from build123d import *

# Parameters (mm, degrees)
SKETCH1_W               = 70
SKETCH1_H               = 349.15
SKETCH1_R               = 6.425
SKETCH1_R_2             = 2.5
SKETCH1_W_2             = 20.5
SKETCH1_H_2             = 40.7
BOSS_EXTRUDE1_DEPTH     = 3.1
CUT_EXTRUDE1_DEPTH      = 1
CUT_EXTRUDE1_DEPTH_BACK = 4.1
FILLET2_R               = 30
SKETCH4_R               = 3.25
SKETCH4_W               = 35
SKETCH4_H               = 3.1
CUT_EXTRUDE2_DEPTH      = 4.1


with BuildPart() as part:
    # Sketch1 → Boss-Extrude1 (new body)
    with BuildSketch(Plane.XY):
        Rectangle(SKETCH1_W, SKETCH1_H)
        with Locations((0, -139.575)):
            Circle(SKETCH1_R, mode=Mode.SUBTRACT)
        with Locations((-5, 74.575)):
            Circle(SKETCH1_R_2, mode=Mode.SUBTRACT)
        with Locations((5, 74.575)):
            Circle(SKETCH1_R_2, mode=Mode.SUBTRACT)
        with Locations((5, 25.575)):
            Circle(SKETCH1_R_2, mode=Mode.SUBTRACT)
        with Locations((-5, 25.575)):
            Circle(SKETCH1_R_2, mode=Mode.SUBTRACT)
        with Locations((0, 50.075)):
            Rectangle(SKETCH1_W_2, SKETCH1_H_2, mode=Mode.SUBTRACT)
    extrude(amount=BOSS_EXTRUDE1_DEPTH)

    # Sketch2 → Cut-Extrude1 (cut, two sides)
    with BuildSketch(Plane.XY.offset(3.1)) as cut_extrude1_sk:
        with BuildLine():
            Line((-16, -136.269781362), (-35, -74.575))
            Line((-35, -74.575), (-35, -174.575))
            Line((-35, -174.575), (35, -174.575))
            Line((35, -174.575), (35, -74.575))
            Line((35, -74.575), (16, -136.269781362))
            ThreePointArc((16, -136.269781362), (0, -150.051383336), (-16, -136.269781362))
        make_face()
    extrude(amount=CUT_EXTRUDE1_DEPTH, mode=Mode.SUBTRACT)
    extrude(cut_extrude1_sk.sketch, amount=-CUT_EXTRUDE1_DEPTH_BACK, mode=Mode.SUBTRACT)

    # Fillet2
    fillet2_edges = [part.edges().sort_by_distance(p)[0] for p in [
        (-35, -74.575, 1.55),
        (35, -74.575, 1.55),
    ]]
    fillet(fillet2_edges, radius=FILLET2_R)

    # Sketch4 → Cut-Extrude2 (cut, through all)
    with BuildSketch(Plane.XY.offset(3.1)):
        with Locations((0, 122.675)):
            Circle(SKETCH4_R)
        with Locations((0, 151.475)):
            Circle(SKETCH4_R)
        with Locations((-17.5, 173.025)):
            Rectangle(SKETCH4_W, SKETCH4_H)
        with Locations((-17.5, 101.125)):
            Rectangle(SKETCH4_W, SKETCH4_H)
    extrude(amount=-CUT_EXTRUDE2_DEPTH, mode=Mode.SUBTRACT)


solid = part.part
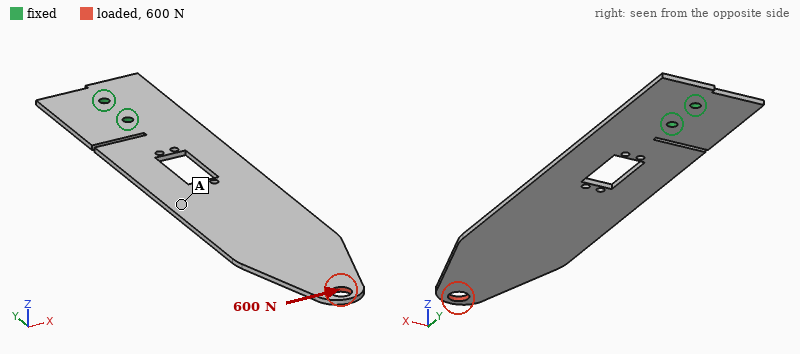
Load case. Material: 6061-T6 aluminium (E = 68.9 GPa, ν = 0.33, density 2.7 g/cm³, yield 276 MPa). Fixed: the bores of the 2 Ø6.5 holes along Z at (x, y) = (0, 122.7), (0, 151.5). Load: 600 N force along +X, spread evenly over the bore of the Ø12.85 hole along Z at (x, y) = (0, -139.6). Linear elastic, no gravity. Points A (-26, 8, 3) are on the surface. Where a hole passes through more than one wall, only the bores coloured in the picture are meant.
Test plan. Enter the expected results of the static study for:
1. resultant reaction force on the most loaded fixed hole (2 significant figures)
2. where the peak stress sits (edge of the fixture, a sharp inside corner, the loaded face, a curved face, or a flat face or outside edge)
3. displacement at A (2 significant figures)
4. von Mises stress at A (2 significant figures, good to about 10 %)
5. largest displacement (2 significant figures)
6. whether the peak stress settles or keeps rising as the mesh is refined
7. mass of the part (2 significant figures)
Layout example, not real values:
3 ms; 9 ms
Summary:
5.5 kN; a sharp inside corner; 1.0 mm; 30 MPa; 2.8 mm; keeps rising; 160 g
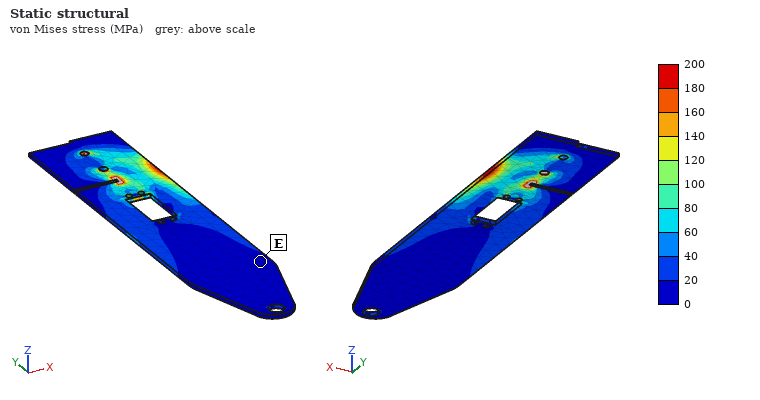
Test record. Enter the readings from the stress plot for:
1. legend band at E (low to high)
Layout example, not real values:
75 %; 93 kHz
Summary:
0 to 20 MPa
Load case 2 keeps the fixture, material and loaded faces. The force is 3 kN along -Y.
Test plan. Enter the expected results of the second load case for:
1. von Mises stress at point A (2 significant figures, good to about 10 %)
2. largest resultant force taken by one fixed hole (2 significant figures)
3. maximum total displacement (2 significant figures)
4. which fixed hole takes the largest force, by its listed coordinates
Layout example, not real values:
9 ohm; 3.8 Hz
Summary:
18 MPa; 2.6 kN; 0.63 mm; (0, 122.7)
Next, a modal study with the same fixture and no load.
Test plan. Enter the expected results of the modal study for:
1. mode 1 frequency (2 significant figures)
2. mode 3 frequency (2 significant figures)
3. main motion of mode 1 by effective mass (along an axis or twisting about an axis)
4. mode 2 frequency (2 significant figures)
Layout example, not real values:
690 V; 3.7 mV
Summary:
33 Hz; 250 Hz; along Z; 220 Hz
